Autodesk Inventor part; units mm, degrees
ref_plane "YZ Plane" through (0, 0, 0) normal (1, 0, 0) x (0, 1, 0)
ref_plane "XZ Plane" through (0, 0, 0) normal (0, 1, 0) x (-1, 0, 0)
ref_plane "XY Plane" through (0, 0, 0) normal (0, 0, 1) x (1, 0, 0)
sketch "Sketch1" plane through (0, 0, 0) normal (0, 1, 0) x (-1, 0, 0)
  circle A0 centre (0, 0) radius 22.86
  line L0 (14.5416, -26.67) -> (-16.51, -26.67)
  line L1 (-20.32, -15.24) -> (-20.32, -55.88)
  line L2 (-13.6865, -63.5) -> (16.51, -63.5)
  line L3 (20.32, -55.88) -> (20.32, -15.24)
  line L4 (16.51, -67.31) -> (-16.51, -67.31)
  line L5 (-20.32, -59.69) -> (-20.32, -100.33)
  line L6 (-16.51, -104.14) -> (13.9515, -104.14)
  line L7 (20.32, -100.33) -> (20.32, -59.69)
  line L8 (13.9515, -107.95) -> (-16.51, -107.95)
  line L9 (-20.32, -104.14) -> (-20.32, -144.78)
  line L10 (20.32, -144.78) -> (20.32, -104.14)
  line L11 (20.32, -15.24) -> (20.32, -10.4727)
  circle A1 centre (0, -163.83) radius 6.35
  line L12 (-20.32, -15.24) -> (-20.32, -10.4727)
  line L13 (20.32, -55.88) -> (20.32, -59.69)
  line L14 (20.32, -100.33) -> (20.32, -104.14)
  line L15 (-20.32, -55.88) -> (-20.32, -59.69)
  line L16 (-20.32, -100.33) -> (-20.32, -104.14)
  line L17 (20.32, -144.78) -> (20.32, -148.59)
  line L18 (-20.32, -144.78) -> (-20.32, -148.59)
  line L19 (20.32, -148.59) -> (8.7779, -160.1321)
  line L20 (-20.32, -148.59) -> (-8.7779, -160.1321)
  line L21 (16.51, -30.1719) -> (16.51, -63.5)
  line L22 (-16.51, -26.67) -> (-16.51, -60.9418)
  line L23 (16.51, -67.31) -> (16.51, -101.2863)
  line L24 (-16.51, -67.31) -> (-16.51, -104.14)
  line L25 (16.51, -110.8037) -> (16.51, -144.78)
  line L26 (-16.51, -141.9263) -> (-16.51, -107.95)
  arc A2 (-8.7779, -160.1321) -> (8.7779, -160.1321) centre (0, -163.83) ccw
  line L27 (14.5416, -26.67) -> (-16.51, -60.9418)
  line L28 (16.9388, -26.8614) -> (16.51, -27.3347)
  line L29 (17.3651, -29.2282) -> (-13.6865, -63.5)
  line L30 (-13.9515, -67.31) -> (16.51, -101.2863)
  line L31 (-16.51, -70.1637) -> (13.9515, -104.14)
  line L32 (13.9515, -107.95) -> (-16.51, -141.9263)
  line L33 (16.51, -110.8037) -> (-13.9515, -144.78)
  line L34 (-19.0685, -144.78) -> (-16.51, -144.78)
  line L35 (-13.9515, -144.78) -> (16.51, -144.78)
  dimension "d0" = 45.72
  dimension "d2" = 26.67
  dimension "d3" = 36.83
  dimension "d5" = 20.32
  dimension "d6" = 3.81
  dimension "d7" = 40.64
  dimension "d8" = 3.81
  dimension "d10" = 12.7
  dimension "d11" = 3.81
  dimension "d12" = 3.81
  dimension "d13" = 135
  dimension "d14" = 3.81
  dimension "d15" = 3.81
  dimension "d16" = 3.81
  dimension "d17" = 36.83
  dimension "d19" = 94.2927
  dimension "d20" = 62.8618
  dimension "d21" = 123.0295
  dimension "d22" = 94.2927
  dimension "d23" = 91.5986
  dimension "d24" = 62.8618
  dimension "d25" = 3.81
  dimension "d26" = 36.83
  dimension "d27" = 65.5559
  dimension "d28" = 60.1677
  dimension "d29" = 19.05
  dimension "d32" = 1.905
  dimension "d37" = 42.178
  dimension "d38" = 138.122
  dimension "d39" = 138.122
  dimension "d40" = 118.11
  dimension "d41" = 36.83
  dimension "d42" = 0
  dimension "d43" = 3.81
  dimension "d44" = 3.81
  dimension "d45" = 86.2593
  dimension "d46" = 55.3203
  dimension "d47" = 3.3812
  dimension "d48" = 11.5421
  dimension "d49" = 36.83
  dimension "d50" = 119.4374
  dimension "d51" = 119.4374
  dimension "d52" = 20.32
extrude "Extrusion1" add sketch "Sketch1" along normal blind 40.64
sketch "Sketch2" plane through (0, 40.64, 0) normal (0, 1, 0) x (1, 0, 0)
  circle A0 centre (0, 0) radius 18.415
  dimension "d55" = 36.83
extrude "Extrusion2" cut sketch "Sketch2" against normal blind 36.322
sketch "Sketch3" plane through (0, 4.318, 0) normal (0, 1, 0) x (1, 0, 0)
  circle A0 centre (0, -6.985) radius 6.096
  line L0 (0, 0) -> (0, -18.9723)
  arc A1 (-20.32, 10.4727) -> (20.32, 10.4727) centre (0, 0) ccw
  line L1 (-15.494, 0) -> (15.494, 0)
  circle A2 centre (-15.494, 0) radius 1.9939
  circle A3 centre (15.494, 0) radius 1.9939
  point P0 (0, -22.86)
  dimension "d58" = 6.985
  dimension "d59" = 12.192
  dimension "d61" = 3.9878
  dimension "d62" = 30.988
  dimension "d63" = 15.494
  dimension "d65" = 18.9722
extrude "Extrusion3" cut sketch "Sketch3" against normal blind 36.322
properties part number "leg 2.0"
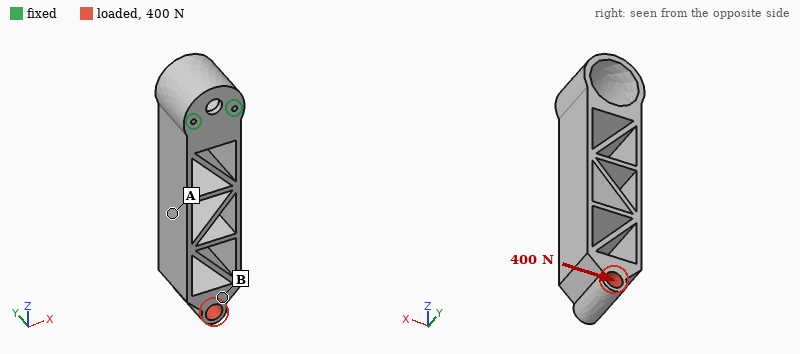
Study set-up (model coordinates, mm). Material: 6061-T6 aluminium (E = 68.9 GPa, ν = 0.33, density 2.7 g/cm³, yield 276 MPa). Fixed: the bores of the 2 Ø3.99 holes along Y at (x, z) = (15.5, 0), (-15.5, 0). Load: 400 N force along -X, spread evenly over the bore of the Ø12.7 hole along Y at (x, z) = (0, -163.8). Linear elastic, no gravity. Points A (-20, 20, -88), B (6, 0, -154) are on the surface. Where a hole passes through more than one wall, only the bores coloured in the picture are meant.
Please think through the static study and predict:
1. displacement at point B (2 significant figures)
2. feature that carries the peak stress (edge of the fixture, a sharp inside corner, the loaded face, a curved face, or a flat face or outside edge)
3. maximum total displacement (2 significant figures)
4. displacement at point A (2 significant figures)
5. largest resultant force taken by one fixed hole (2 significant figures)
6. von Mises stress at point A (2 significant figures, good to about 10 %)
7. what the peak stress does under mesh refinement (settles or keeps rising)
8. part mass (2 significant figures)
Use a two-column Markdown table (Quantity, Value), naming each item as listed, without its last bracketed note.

| Quantity | Value |
|---|---|
| displacement at point B | 0.14 mm |
| feature that carries the peak stress | edge of the fixture |
| maximum total displacement | 0.17 mm |
| displacement at point A | 0.068 mm |
| largest resultant force taken by one fixed hole | 2.0 kN |
| von Mises stress at point A | 6.8 MPa |
| what the peak stress does under mesh refinement | keeps rising |
| part mass | 360 g |
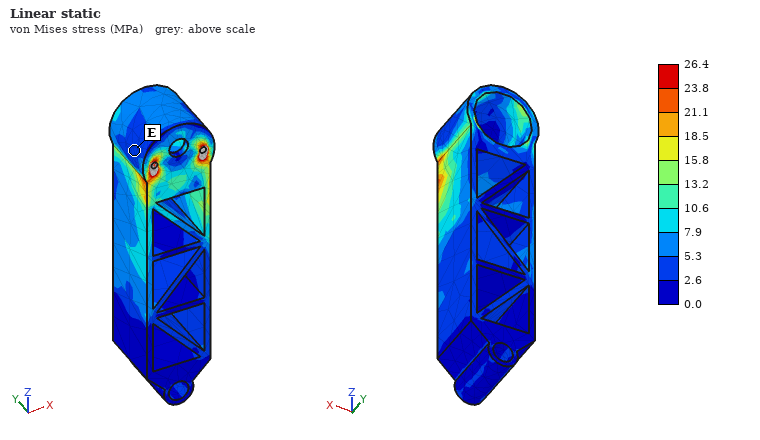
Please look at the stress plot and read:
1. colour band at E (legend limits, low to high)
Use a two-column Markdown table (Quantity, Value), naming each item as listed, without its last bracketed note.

| Quantity | Value |
|---|---|
| colour band at E | 2.6 to 5.3 MPa |
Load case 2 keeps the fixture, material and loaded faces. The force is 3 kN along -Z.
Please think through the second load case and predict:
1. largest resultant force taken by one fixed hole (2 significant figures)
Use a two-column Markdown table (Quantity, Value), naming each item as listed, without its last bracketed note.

| Quantity | Value |
|---|---|
| largest resultant force taken by one fixed hole | 1.5 kN |
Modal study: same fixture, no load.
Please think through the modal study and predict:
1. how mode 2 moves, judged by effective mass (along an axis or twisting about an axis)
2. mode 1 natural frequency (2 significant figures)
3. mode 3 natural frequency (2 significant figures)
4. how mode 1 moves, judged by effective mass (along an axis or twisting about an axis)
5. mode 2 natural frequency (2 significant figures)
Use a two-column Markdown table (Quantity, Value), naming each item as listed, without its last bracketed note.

| Quantity | Value |
|---|---|
| how mode 2 moves, judged by effective mass | along X |
| mode 1 natural frequency | 240 Hz |
| mode 3 natural frequency | 2300 Hz |
| how mode 1 moves, judged by effective mass | along Y |
| mode 2 natural frequency | 810 Hz |
